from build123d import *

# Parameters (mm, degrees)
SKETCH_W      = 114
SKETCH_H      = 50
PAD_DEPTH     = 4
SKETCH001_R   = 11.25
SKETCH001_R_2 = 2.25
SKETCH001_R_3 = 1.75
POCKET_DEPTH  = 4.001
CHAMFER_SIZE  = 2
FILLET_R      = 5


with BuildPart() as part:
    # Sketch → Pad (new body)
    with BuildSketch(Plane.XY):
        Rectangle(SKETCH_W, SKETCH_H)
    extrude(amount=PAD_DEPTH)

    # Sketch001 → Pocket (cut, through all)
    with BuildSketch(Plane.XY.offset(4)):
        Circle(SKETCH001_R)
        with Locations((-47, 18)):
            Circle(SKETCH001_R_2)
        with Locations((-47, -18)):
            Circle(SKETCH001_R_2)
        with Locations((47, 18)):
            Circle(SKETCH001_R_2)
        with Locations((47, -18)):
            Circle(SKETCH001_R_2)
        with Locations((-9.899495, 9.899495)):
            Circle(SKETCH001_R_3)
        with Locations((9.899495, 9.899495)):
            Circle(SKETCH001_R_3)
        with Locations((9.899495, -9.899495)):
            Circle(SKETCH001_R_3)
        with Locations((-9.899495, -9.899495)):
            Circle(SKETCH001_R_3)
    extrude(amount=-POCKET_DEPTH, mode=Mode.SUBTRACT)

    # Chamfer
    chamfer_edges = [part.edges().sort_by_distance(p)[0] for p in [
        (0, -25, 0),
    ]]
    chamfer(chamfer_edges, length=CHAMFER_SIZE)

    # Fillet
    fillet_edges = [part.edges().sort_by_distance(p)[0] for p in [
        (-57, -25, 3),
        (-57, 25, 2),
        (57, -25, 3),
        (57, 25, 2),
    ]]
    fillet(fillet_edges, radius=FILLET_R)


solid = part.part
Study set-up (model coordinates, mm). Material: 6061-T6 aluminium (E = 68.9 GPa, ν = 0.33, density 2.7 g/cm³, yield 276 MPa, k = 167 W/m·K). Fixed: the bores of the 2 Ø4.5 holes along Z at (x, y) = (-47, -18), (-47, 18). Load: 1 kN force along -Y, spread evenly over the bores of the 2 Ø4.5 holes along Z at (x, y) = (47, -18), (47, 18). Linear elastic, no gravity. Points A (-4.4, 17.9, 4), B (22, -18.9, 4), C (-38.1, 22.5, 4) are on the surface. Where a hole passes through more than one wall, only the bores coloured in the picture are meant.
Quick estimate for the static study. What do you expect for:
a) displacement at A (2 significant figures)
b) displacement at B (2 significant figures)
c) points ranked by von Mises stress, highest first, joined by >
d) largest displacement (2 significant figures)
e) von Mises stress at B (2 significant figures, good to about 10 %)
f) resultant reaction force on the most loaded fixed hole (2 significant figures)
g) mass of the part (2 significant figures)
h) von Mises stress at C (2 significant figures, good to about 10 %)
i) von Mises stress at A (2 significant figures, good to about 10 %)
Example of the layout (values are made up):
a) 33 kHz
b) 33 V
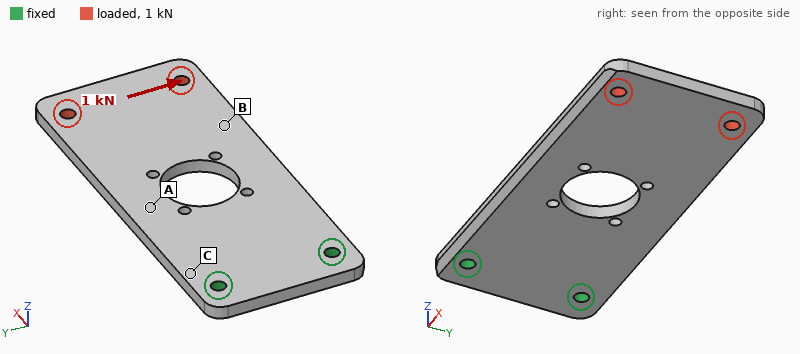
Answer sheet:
a) 0.051 mm
b) 0.11 mm
c) C > A > B
d) 0.17 mm
e) 12 MPa
f) 2.6 kN
g) 55 g
h) 46 MPa
i) 34 MPa
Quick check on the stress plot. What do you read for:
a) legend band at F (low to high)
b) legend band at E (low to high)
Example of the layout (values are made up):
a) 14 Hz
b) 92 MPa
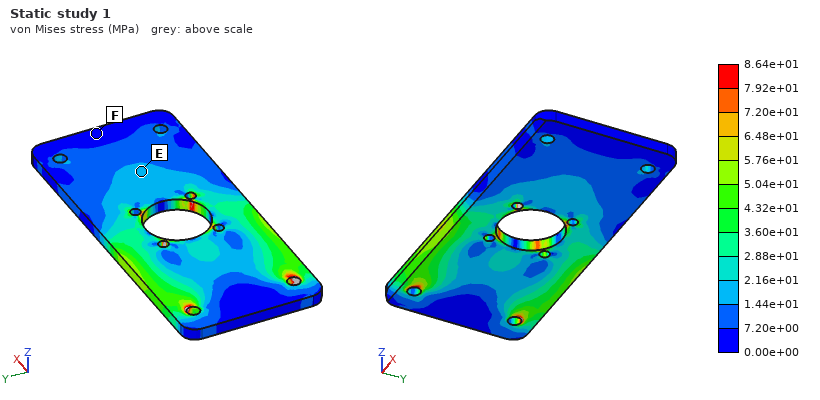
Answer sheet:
a) 0.00e+00 to 7.20e+00 MPa
b) 1.44e+01 to 2.16e+01 MPa
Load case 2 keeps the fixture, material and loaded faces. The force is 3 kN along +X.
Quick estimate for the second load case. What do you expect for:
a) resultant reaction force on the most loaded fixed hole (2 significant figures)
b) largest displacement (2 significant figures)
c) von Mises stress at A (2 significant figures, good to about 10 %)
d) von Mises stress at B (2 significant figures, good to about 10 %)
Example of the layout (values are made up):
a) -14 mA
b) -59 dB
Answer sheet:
a) 1.5 kN
b) 42 µm
c) 25 MPa
d) 23 MPa
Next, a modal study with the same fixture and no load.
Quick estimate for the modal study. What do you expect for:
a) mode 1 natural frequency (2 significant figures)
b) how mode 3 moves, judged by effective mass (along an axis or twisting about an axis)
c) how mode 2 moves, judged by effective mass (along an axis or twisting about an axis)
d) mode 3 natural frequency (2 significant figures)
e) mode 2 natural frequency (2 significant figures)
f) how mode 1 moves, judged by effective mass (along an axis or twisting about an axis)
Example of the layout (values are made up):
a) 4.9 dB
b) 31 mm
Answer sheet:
a) 290 Hz
b) along Z
c) twisting about X
d) 1800 Hz
e) 1200 Hz
f) along Z
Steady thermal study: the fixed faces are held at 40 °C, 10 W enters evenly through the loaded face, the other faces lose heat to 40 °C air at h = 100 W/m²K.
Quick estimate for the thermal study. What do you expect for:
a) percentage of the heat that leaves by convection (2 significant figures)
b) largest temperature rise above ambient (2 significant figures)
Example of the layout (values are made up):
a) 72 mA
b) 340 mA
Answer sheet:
a) 76 %
b) 16 K
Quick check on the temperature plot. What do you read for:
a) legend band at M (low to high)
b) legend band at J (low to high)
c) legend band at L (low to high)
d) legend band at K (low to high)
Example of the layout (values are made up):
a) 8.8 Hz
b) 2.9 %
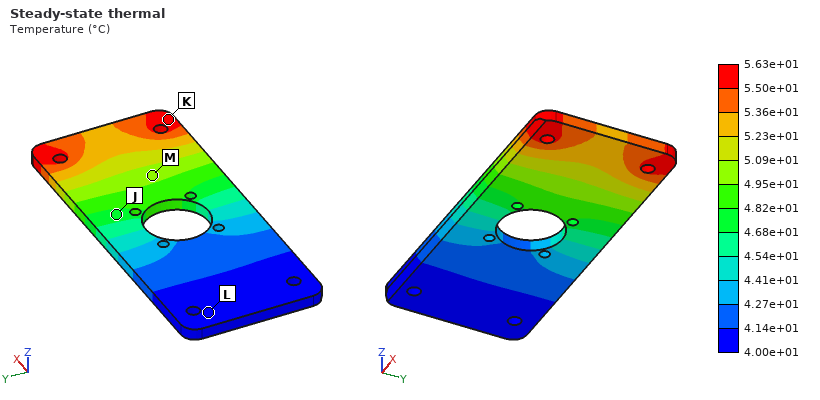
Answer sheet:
a) 4.95e+01 to 5.09e+01 °C
b) 4.68e+01 to 4.82e+01 °C
c) 4.00e+01 to 4.14e+01 °C
d) 5.50e+01 to 5.63e+01 °C
